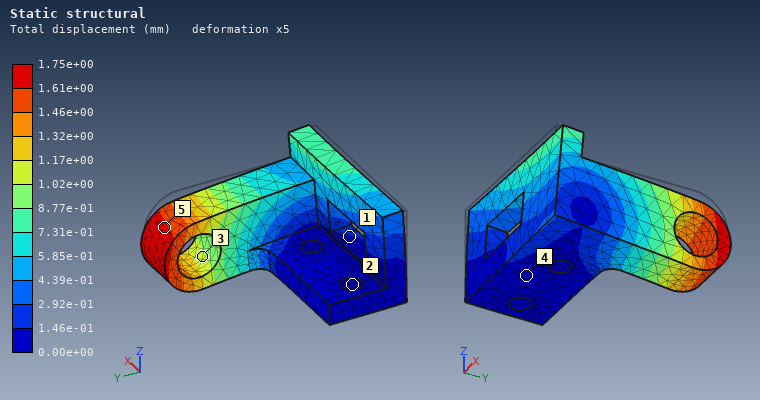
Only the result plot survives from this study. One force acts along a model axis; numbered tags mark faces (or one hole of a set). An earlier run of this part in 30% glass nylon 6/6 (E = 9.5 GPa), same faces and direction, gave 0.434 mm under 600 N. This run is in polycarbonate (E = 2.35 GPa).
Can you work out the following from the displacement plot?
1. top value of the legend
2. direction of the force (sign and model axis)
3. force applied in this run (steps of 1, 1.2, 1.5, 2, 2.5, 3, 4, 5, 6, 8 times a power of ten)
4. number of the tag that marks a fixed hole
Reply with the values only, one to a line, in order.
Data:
1.75e+00 mm
-Z
600 N
2
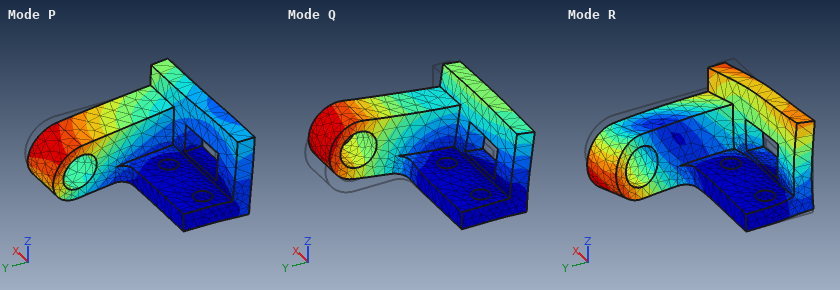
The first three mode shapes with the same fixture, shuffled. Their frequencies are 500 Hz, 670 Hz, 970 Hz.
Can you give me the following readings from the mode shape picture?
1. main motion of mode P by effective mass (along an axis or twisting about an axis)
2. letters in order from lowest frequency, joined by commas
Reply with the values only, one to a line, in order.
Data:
along X
Q, P, R
